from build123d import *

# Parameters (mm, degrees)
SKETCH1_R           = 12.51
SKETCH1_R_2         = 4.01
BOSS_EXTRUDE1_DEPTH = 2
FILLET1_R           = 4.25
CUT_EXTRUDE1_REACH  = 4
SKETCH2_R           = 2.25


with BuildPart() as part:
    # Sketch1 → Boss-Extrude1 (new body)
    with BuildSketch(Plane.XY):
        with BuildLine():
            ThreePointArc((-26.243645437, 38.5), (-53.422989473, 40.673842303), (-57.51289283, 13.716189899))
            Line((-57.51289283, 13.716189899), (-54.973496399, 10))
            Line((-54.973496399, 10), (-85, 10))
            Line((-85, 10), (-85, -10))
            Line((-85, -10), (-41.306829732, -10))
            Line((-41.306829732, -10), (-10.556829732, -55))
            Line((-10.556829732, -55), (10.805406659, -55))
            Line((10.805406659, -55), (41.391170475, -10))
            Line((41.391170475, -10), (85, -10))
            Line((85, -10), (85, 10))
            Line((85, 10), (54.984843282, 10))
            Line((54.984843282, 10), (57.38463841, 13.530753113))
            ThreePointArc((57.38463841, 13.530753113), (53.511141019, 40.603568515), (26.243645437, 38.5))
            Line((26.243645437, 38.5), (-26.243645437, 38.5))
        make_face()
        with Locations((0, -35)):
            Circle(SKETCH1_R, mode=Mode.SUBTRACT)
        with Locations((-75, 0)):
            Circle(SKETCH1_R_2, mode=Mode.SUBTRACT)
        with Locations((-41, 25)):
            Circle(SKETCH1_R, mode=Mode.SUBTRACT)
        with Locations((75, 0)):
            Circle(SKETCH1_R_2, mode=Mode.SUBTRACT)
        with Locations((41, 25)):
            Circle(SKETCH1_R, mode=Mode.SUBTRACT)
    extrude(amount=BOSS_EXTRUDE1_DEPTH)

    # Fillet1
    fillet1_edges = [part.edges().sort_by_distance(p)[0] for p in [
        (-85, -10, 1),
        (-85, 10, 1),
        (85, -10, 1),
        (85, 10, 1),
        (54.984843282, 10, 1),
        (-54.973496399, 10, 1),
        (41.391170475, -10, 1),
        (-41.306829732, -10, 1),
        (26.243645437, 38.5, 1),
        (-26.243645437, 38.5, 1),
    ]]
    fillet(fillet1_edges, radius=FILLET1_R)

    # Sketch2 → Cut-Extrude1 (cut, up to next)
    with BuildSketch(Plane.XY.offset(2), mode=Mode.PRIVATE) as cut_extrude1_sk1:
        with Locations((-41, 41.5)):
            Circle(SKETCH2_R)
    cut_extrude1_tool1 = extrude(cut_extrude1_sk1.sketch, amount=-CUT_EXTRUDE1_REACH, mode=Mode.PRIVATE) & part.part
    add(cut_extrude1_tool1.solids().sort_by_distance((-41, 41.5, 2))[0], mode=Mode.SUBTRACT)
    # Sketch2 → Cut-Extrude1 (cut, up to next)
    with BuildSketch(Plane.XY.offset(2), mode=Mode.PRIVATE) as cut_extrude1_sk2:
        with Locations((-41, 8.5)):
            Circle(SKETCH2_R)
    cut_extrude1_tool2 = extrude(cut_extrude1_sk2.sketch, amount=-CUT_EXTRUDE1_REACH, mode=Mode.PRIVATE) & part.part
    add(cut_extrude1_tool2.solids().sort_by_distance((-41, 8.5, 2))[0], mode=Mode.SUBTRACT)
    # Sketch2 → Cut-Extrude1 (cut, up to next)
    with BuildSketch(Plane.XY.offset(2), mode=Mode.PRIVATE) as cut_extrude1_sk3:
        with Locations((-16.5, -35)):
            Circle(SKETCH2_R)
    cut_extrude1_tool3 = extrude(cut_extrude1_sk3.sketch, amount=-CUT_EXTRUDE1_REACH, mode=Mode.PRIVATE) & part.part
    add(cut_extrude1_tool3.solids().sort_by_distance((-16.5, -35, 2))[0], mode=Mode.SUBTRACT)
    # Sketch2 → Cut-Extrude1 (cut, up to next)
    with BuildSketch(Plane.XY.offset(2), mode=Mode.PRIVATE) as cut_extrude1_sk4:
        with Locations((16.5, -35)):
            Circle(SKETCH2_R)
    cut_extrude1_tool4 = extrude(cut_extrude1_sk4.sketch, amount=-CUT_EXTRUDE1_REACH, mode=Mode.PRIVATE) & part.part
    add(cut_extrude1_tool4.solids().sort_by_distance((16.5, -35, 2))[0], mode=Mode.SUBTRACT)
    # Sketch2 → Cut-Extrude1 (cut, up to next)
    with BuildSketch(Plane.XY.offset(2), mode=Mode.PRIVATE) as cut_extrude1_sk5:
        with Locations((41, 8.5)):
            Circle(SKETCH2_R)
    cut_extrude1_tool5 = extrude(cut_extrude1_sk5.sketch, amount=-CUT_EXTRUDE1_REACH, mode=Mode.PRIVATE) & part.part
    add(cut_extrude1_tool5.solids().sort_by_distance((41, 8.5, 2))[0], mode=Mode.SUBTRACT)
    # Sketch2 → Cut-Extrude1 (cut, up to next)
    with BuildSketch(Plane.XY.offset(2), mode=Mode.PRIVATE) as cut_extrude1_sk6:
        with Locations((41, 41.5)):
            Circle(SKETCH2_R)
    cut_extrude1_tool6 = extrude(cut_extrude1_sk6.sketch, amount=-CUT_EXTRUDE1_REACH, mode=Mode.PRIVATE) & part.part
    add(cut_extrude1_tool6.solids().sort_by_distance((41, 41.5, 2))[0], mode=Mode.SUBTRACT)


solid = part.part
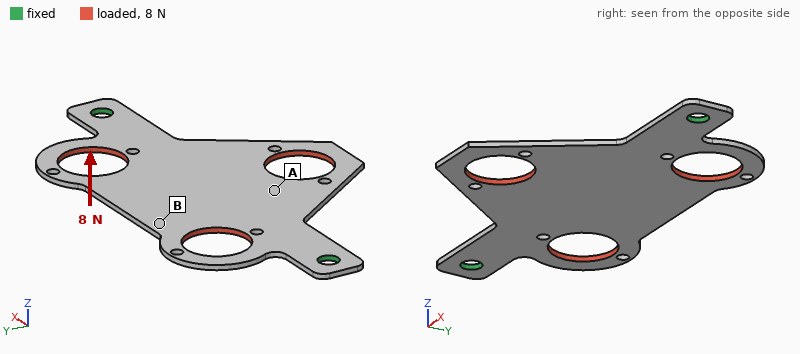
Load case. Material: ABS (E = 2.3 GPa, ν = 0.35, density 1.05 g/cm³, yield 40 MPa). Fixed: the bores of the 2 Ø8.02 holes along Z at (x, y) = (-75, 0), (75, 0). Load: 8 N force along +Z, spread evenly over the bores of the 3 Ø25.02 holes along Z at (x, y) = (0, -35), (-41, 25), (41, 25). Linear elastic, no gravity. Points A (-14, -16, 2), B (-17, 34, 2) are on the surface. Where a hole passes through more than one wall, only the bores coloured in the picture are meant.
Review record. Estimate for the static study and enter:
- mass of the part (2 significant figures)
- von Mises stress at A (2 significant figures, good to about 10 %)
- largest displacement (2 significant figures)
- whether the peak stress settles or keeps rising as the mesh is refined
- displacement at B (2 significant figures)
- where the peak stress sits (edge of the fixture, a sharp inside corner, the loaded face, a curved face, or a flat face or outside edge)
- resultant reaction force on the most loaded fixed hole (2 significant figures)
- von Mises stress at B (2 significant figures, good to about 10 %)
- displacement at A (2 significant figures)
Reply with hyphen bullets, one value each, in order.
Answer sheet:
- 16 g
- 2.1 MPa
- 2.3 mm
- keeps rising
- 1.5 mm
- edge of the fixture
- 4.0 N
- 1.0 MPa
- 1.4 mm
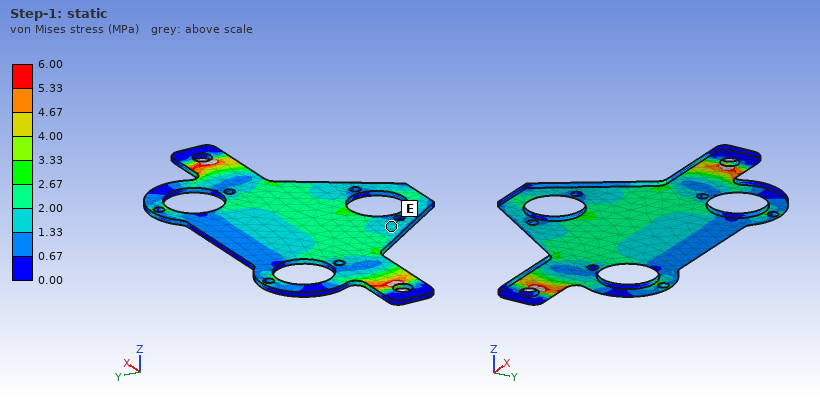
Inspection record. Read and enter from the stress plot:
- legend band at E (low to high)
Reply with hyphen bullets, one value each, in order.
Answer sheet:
- 1.33 to 2.00 MPa
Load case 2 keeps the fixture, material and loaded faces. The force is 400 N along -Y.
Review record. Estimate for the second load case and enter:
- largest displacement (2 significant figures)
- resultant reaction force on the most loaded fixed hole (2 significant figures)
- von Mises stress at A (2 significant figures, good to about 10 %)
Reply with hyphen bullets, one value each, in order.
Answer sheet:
- 0.59 mm
- 200 N
- 2.9 MPa
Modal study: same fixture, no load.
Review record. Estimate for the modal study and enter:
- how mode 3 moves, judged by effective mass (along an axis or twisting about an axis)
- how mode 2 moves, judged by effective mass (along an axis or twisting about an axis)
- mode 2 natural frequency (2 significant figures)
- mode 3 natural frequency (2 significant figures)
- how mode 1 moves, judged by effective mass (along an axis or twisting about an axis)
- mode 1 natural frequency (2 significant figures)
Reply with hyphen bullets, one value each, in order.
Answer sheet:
- twisting about Y
- along Z
- 100 Hz
- 270 Hz
- along Z
- 95 Hz
